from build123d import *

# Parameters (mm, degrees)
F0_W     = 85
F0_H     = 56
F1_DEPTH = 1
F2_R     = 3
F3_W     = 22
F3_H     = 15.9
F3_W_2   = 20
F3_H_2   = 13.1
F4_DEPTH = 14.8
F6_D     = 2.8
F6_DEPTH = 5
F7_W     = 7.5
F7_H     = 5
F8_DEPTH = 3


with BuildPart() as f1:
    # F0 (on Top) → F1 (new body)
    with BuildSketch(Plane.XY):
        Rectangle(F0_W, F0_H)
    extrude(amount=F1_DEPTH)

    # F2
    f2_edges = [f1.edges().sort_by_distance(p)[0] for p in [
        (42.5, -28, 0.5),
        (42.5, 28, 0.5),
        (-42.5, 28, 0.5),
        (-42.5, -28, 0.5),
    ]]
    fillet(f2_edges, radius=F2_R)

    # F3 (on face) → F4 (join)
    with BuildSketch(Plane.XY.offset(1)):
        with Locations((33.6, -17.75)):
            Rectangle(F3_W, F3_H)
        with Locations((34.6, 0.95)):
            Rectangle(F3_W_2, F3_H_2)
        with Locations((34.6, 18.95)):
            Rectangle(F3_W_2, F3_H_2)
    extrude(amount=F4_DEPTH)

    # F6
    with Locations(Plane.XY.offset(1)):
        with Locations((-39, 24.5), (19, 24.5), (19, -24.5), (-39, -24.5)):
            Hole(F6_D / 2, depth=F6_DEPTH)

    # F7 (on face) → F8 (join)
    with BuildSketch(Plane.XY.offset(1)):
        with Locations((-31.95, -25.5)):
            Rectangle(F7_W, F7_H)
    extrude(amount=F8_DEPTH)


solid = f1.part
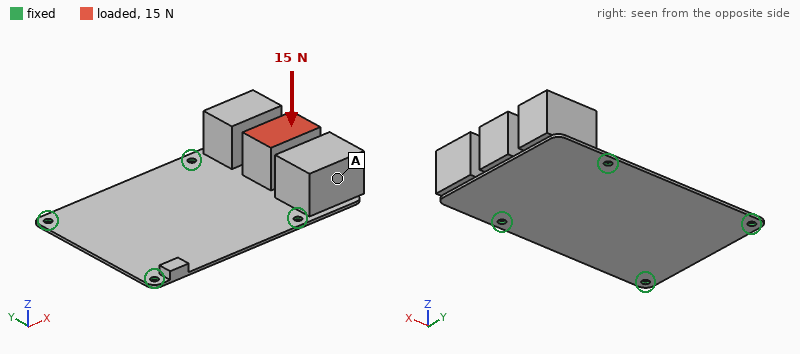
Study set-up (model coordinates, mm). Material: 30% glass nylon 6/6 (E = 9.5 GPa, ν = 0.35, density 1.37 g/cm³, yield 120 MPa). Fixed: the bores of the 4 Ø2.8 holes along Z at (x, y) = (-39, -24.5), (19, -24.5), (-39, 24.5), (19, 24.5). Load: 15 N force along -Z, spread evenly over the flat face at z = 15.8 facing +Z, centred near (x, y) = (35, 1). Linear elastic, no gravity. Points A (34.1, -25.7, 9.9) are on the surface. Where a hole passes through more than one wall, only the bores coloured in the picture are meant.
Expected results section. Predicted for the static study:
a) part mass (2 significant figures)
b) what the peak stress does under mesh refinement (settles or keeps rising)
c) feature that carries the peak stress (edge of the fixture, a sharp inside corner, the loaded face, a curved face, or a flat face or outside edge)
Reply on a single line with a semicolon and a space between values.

24 g; keeps rising; edge of the fixture
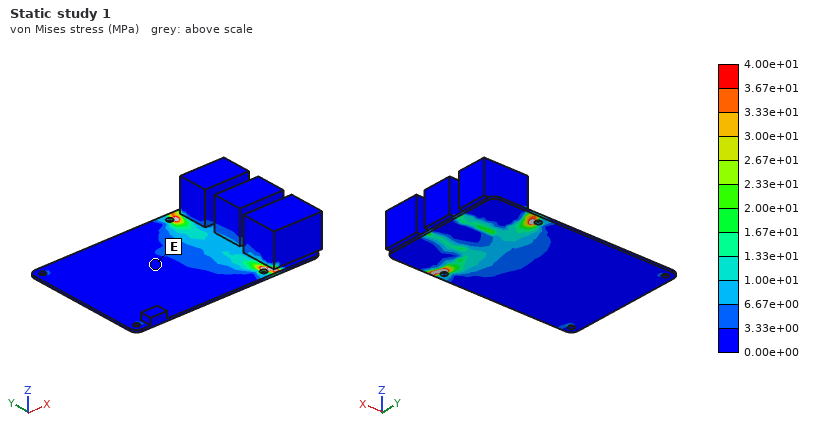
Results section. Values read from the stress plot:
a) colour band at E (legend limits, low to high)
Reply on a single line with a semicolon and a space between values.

0.00e+00 to 3.33e+00 MPa
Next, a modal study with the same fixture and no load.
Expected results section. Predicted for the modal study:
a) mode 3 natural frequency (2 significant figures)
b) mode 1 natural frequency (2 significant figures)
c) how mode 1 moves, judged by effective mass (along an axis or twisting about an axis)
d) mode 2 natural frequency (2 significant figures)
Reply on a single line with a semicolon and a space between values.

710 Hz; 170 Hz; along Z; 540 Hz
